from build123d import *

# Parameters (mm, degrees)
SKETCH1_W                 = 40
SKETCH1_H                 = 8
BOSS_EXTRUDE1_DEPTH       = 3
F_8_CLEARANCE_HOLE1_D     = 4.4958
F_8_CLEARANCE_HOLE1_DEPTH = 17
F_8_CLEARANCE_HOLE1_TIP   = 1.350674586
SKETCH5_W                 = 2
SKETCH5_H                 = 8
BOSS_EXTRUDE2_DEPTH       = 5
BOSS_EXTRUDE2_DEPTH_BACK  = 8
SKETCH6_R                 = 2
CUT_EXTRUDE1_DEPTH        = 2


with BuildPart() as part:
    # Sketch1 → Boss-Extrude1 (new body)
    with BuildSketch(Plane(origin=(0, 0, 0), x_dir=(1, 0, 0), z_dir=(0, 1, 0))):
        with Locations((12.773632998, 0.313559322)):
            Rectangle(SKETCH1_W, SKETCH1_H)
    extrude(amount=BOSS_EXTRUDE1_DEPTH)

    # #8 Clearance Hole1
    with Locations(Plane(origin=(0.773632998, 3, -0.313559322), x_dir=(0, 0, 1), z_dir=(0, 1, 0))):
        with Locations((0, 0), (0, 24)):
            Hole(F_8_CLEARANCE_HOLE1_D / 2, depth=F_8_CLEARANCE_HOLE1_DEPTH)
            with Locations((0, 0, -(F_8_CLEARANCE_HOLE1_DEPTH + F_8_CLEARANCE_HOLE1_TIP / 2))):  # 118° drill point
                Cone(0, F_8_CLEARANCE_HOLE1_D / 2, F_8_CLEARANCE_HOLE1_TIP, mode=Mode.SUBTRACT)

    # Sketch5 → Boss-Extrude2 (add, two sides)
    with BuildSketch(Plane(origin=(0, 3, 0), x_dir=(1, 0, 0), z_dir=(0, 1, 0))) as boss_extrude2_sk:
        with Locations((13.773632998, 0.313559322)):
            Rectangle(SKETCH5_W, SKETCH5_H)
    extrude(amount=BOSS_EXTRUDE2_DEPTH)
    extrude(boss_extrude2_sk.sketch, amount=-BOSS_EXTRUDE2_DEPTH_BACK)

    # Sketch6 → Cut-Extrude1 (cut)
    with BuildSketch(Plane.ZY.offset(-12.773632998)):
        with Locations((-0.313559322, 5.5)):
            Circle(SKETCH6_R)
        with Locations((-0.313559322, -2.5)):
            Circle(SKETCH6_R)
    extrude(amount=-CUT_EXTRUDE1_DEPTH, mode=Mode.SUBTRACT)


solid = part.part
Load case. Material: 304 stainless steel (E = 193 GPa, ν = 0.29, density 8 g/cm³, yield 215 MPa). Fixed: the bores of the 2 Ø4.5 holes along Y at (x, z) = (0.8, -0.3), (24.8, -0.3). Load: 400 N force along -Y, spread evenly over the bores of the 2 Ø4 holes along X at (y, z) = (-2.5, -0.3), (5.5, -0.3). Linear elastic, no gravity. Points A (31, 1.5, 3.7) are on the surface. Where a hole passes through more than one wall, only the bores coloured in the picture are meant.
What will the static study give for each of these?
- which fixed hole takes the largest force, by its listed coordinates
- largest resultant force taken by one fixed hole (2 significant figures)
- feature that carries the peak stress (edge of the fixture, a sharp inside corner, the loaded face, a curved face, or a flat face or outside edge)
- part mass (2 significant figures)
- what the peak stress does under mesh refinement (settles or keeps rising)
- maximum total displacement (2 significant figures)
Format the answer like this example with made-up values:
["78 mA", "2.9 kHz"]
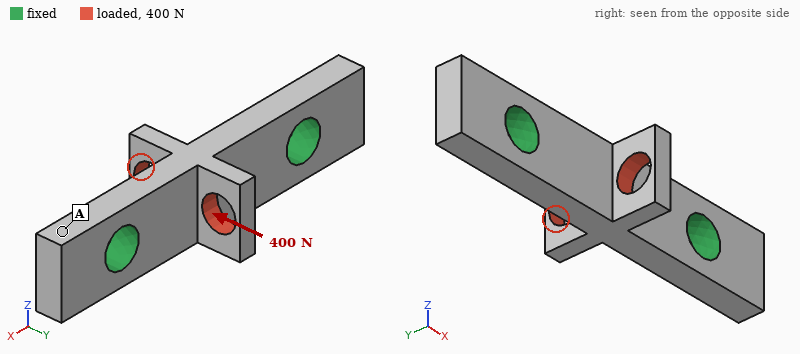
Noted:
["(24.8, -0.3)", "230 N", "edge of the fixture", "7.8 g", "keeps rising", "7.5 µm"]
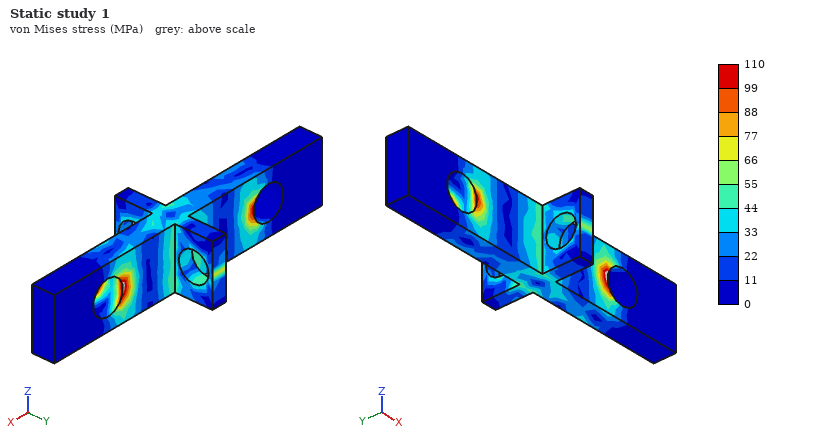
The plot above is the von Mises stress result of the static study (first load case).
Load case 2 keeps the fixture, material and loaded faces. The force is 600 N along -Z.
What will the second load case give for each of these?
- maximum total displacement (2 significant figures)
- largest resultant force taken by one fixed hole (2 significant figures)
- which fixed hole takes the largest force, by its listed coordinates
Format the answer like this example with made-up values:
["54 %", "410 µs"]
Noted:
["9.2 µm", "340 N", "(24.8, -0.3)"]
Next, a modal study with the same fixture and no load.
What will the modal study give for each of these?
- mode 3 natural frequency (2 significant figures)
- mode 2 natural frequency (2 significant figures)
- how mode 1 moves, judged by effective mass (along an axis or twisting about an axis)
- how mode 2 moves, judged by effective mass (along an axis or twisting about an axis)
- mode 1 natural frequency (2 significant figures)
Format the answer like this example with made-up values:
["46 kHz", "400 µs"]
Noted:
["37 kHz", "27 kHz", "along Y", "twisting about X", "26 kHz"]
